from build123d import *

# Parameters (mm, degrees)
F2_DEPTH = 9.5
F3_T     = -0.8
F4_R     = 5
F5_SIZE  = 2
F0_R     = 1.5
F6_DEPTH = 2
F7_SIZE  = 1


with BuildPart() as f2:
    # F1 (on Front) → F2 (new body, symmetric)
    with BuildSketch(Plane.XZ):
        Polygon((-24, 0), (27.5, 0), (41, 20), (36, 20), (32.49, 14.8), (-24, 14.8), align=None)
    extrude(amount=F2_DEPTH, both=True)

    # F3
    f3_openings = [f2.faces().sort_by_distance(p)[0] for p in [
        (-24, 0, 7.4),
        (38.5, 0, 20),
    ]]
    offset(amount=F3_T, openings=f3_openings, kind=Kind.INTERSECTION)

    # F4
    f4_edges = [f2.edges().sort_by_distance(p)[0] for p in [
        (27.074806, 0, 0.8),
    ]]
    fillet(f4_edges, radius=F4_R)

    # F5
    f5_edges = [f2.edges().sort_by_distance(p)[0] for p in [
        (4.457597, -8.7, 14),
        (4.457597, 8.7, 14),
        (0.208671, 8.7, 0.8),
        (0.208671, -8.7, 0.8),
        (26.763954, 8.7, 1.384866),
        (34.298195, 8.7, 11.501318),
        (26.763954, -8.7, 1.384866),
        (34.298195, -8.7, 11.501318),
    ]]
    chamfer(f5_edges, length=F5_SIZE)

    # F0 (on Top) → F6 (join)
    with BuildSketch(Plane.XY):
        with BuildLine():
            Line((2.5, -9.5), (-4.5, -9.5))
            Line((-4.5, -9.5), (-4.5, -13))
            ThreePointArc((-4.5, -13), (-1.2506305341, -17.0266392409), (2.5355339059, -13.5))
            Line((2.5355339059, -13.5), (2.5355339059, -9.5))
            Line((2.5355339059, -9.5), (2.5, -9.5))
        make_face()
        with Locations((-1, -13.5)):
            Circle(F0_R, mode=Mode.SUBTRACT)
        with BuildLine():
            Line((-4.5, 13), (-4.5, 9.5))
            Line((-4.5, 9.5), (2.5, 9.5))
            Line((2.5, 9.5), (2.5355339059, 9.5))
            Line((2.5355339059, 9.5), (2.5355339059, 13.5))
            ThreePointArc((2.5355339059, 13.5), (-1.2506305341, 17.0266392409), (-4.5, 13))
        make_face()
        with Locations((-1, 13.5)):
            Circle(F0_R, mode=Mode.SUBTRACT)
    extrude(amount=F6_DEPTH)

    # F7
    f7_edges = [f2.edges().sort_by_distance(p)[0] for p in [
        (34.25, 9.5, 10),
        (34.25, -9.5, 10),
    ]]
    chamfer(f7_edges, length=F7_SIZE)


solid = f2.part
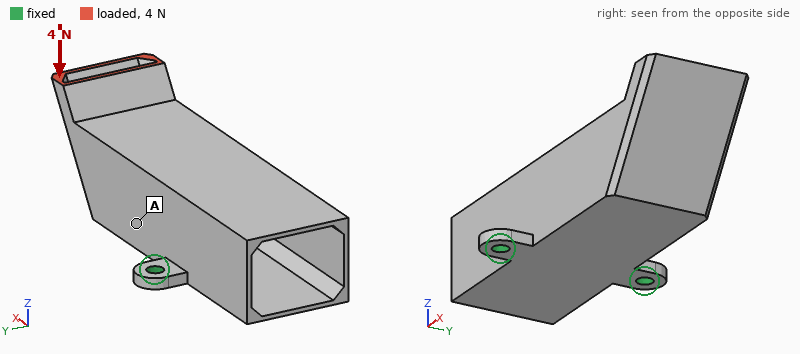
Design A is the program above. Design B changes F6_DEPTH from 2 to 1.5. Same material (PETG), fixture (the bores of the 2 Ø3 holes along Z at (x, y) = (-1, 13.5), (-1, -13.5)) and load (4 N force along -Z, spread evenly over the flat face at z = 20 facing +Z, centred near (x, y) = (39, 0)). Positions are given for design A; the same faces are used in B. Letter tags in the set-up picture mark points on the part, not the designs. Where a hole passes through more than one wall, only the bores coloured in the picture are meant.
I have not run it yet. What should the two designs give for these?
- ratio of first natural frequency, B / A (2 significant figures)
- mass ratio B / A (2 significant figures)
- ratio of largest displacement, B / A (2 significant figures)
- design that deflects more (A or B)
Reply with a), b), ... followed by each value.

a) 0.75
b) 0.99
c) 1.7
d) B
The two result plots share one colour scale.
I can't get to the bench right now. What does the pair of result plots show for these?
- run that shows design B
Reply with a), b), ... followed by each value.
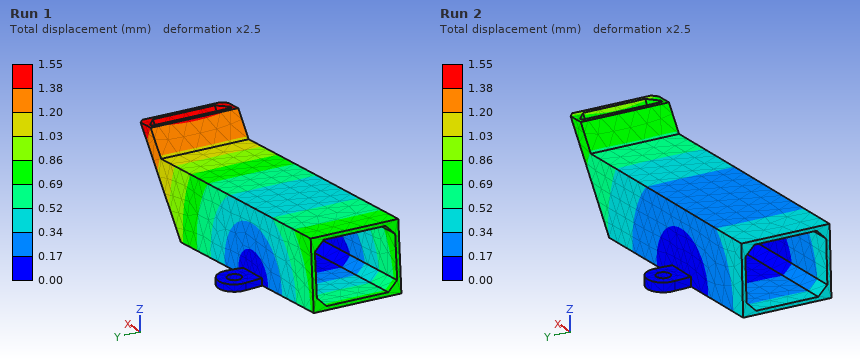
a) Run 1
